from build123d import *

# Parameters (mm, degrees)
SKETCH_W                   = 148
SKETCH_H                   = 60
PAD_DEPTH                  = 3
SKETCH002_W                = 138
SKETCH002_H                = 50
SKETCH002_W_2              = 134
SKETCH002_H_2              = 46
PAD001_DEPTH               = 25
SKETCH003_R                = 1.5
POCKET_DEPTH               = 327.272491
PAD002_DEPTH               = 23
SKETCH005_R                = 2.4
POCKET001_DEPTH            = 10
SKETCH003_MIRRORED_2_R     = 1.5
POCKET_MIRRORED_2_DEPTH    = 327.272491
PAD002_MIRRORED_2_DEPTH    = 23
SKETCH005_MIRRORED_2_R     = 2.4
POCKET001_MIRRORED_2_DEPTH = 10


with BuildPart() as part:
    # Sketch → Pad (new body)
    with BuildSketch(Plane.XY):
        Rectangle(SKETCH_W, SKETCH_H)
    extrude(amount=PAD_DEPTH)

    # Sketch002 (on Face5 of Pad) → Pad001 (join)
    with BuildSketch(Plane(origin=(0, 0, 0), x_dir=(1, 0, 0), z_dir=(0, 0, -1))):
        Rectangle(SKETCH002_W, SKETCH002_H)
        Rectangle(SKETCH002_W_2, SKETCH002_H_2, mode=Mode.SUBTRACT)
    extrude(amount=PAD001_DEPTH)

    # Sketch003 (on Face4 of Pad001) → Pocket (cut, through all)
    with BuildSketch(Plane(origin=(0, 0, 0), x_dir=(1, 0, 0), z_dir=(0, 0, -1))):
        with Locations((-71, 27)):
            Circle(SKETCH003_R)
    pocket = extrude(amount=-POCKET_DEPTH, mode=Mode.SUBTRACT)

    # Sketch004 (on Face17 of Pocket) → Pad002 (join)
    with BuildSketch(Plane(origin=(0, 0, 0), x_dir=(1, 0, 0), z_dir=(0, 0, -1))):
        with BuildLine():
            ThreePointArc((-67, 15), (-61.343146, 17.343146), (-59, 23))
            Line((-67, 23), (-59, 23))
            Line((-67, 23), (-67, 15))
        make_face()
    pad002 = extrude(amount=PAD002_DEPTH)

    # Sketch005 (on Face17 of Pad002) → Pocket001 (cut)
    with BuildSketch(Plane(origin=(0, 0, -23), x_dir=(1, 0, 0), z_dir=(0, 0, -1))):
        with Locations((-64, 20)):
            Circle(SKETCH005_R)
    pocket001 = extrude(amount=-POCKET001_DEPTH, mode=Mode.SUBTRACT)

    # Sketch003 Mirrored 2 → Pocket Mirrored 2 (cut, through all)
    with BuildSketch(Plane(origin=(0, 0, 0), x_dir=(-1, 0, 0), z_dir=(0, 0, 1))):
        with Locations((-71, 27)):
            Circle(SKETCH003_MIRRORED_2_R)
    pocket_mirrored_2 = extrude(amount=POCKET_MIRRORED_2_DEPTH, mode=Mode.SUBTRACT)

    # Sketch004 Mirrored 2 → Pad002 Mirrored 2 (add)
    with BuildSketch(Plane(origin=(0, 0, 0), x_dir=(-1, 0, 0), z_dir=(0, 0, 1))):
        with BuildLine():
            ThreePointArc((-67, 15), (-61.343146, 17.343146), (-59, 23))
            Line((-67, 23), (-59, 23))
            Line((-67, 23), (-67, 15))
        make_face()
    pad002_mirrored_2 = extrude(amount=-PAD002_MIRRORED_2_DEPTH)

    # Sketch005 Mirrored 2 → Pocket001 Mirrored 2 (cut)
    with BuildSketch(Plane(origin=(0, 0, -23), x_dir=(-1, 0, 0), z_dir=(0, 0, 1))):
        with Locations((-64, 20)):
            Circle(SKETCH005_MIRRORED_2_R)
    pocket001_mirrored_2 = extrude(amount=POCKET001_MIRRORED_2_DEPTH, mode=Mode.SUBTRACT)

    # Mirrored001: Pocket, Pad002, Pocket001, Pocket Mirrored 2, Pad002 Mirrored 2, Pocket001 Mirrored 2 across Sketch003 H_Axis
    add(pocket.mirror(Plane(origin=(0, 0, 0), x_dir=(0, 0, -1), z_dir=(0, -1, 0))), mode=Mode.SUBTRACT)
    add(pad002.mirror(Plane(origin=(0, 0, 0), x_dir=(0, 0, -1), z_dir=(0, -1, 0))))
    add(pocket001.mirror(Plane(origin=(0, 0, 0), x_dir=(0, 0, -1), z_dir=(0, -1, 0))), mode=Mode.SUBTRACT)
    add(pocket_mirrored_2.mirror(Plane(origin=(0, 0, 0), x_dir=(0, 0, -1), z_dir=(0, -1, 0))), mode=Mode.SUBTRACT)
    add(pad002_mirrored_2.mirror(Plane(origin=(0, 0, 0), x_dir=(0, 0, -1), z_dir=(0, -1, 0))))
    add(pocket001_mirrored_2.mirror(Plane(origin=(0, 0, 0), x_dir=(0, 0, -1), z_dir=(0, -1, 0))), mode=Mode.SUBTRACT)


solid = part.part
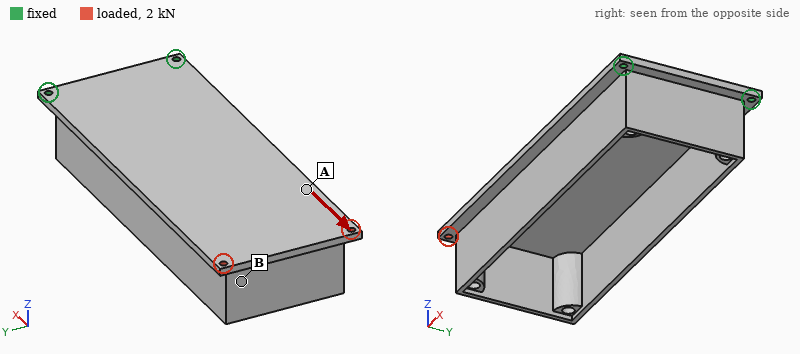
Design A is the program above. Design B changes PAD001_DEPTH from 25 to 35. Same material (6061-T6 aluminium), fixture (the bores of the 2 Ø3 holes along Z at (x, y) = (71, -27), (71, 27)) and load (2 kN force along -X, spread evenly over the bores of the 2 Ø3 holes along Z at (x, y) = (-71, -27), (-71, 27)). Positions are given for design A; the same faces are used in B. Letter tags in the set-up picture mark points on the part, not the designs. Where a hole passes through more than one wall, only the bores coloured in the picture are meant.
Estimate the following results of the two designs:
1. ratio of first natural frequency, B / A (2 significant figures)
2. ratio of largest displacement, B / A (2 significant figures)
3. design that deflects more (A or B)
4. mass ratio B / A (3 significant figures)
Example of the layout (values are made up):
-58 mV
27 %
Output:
0.93
0.83
A
1.15
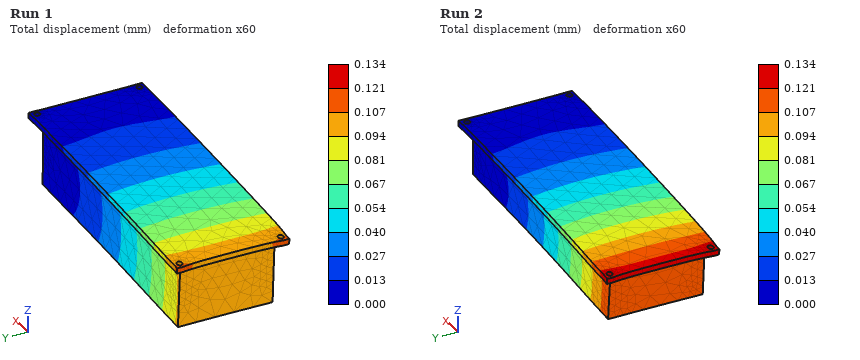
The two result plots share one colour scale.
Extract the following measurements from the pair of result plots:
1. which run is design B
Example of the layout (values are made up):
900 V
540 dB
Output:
Run 1
